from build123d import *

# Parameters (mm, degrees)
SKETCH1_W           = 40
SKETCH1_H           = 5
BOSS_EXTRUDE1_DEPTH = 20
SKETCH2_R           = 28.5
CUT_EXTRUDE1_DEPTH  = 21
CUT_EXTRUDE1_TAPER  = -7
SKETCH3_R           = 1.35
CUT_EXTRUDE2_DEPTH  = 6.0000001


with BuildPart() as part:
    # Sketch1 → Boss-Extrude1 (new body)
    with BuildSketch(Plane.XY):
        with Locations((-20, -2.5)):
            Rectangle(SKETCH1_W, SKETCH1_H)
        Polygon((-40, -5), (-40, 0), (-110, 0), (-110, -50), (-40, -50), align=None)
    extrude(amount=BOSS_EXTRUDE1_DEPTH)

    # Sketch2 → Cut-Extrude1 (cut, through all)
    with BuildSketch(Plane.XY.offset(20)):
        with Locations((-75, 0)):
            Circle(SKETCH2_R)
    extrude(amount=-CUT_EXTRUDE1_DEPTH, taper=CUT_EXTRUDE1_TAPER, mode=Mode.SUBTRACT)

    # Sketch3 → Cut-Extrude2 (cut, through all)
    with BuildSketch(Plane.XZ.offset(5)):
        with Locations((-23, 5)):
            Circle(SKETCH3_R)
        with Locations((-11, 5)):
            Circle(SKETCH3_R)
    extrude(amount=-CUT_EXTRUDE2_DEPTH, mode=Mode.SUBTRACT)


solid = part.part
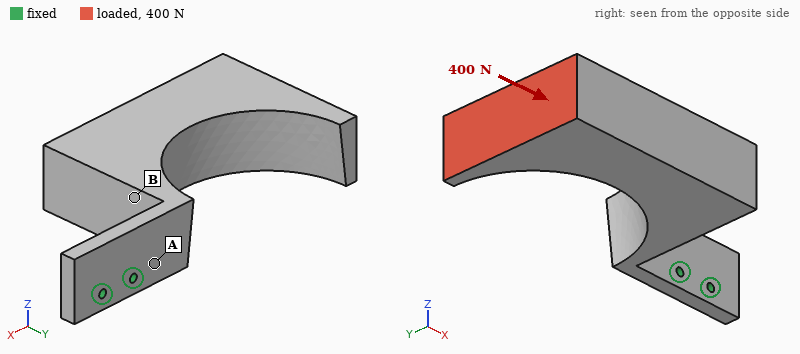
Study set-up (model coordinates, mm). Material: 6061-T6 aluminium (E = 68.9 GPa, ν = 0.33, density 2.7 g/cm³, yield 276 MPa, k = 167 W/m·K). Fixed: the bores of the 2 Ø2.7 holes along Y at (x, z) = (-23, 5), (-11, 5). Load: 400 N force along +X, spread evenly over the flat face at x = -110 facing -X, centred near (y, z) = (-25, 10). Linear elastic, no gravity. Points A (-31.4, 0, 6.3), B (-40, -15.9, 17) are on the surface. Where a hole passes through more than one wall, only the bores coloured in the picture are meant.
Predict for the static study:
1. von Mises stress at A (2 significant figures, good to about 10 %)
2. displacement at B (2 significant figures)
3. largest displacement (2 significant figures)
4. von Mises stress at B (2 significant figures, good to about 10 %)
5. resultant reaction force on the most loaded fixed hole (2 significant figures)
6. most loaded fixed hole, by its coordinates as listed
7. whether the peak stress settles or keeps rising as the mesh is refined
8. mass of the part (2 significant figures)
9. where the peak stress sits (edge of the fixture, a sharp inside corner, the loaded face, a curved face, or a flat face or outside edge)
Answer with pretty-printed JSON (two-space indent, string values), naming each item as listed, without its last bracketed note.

{
  "von Mises stress at A": "100 MPa",
  "displacement at B": "0.22 mm",
  "largest displacement": "1.4 mm",
  "von Mises stress at B": "16 MPa",
  "resultant reaction force on the most loaded fixed hole": "450 N",
  "most loaded fixed hole, by its coordinates as listed": "(-23, 5)",
  "whether the peak stress settles or keeps rising as the mesh is refined": "keeps rising",
  "mass of the part": "120 g",
  "where the peak stress sits": "edge of the fixture"
}
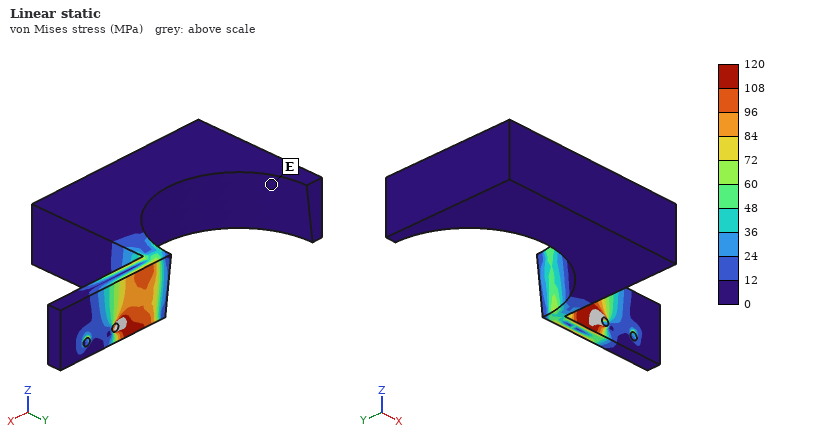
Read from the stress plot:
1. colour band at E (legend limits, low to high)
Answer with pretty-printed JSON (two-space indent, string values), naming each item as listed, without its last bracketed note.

{
  "colour band at E": "0 to 12 MPa"
}
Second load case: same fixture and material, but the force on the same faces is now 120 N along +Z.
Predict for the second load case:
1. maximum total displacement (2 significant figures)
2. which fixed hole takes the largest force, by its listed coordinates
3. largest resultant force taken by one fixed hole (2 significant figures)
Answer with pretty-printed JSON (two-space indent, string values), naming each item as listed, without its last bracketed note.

{
  "maximum total displacement": "0.34 mm",
  "which fixed hole takes the largest force, by its listed coordinates": "(-23, 5)",
  "largest resultant force taken by one fixed hole": "860 N"
}
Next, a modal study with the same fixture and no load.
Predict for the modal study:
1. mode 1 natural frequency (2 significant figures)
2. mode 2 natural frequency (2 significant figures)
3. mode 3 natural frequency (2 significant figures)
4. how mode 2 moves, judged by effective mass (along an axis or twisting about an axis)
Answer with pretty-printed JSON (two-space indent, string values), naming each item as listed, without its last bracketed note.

{
  "mode 1 natural frequency": "190 Hz",
  "mode 2 natural frequency": "380 Hz",
  "mode 3 natural frequency": "920 Hz",
  "how mode 2 moves, judged by effective mass": "along Z"
}
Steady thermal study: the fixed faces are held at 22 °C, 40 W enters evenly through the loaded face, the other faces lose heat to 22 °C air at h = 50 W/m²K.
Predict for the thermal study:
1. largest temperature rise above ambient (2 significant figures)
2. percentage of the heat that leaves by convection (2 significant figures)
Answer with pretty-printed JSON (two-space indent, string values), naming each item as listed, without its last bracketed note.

{
  "largest temperature rise above ambient": "71 K",
  "percentage of the heat that leaves by convection": "55 %"
}
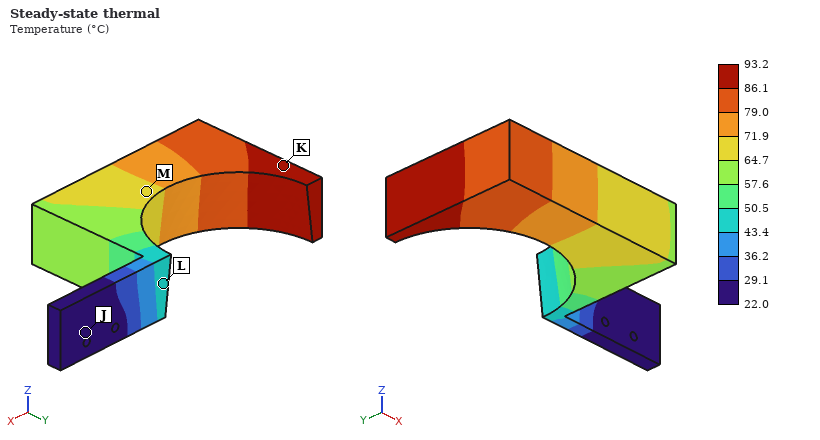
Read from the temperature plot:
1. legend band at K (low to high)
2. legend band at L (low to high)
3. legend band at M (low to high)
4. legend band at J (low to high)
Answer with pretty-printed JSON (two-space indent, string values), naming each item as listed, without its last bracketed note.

{
  "legend band at K": "86.1 to 93.2 °C",
  "legend band at L": "43.4 to 50.5 °C",
  "legend band at M": "64.7 to 71.9 °C",
  "legend band at J": "22.0 to 29.1 °C"
}
